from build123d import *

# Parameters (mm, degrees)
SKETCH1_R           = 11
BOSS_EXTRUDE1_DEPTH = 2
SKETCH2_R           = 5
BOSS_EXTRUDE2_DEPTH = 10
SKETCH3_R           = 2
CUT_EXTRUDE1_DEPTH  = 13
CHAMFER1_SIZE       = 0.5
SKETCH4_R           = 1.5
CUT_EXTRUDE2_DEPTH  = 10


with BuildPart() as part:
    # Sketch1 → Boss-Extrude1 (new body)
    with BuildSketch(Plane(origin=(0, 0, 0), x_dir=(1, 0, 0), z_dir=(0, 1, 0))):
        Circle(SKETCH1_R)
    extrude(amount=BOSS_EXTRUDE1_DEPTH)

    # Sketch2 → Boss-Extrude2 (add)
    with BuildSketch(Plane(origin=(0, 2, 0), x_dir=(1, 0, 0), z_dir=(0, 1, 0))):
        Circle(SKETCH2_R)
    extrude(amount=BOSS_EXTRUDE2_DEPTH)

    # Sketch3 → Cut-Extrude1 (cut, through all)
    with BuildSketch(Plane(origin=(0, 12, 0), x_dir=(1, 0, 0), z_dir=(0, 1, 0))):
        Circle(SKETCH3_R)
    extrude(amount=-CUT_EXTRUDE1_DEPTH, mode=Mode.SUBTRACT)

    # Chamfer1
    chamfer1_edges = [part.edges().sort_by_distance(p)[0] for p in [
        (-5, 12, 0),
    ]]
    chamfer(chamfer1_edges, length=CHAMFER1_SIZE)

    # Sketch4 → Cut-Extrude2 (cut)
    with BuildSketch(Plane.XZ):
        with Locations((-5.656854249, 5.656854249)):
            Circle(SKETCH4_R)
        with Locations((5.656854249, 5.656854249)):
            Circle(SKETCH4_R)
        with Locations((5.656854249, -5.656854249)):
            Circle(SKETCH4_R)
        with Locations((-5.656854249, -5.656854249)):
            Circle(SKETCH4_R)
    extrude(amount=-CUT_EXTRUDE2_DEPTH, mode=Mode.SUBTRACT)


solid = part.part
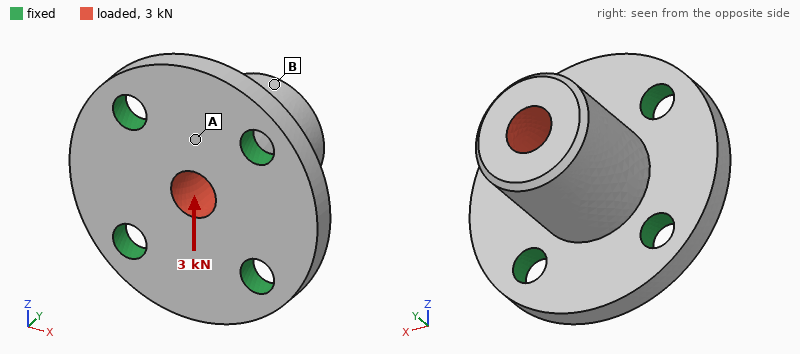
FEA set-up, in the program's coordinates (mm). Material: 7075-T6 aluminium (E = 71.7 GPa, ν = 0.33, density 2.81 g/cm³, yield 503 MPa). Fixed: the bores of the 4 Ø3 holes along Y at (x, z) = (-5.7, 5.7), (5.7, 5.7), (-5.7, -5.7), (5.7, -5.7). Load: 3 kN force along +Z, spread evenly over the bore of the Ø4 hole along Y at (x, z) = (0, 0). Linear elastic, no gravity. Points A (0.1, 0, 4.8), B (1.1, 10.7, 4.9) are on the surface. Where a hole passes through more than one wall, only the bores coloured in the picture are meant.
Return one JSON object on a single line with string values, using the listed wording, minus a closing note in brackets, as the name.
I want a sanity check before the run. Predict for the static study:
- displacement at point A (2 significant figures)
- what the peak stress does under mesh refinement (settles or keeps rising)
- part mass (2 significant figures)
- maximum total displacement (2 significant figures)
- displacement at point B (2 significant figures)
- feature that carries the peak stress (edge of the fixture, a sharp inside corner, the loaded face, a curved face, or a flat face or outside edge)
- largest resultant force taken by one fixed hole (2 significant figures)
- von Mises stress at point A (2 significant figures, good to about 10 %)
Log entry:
{"displacement at point A": "14 µm", "what the peak stress does under mesh refinement": "keeps rising", "part mass": "3.8 g", "maximum total displacement": "57 µm", "displacement at point B": "52 µm", "feature that carries the peak stress": "edge of the fixture", "largest resultant force taken by one fixed hole": "1.1 kN", "von Mises stress at point A": "120 MPa"}
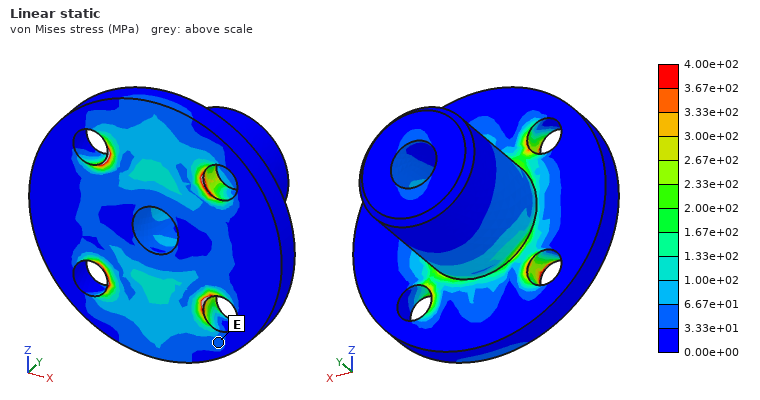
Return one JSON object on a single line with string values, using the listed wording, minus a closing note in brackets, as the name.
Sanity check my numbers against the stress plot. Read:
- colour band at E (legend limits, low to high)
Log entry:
{"colour band at E": "3.33e+01 to 6.67e+01 MPa"}
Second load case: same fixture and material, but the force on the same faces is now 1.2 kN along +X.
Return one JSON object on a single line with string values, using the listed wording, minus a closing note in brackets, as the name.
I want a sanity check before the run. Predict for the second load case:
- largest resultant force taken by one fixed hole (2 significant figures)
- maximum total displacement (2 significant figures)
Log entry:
{"largest resultant force taken by one fixed hole": "450 N", "maximum total displacement": "23 µm"}
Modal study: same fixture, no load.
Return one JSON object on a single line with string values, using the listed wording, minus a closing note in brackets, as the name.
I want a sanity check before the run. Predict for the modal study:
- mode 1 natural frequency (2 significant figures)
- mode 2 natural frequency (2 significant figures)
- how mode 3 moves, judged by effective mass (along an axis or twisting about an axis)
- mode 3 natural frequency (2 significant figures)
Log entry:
{"mode 1 natural frequency": "29 kHz", "mode 2 natural frequency": "29 kHz", "how mode 3 moves, judged by effective mass": "along Y", "mode 3 natural frequency": "48 kHz"}
